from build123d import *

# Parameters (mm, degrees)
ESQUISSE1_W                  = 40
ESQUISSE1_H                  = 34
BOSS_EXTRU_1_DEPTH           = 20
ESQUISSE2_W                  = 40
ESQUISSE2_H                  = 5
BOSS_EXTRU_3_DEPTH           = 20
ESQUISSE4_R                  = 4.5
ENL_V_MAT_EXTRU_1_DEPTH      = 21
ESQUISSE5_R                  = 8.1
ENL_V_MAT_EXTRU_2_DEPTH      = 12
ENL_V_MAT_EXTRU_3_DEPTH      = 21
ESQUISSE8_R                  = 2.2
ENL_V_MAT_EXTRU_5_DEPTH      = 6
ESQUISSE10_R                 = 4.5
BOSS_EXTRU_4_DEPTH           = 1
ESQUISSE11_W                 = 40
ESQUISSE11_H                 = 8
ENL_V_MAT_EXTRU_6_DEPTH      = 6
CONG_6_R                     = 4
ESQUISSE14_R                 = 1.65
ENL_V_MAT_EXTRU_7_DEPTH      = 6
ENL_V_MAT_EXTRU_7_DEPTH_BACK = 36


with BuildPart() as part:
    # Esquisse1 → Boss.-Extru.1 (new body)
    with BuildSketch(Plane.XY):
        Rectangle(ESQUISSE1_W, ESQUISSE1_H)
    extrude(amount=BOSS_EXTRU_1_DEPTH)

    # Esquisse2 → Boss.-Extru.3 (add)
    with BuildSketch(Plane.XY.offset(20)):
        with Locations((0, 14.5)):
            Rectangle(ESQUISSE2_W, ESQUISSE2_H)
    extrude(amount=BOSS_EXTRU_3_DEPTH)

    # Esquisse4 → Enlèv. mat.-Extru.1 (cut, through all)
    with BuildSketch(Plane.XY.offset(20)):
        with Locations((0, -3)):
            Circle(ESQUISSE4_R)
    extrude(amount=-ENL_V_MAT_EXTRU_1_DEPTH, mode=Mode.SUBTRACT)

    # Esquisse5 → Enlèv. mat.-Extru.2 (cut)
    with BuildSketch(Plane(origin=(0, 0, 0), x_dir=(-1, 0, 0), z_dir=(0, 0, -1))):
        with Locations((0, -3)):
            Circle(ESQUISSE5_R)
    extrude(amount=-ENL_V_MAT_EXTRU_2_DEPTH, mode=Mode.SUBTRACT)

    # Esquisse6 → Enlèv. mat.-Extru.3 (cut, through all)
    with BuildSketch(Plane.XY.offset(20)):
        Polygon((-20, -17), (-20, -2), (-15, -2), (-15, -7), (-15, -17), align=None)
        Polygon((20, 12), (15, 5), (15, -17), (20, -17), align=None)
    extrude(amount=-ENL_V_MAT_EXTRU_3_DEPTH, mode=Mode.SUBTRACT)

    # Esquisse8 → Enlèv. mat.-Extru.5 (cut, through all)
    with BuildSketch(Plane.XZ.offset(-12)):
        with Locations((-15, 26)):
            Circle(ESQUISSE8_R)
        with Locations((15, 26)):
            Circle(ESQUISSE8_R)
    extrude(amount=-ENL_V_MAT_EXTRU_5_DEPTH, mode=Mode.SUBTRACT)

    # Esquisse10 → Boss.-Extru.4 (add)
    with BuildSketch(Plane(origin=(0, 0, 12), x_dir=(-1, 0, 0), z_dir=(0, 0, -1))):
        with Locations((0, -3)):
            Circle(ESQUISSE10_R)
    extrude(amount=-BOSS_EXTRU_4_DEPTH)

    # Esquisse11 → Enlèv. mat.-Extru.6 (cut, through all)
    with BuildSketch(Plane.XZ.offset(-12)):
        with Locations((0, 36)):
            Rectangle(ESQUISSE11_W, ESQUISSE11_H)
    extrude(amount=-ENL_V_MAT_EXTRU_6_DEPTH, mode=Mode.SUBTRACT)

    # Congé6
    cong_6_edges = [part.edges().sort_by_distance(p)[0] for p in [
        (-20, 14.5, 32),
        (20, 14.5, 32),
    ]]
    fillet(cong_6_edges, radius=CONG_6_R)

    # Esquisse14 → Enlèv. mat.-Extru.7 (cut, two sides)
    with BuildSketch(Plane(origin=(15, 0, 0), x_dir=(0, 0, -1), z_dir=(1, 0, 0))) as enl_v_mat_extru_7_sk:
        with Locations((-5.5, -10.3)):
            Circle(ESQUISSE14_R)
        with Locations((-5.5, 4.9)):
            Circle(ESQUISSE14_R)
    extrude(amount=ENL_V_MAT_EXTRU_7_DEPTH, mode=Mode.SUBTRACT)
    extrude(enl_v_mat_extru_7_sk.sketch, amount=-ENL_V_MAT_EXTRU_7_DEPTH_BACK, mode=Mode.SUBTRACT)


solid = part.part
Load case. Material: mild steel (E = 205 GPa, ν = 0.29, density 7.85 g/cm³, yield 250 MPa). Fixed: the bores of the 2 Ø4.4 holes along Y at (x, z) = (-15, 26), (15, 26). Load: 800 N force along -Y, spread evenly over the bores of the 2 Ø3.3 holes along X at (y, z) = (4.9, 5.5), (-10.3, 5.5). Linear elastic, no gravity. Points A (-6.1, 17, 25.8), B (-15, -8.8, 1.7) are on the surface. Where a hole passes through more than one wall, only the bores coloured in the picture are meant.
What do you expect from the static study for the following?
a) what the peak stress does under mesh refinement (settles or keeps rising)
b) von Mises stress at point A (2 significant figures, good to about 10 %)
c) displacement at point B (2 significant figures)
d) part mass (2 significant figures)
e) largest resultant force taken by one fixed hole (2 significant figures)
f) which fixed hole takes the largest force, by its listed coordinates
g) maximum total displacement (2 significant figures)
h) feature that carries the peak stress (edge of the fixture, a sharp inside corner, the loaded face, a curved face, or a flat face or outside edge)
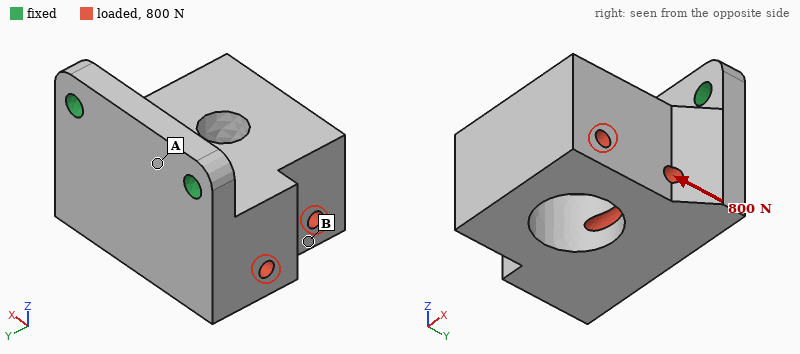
keeps rising
32 MPa
45 µm
170 g
440 N
(-15, 26)
56 µm
edge of the fixture
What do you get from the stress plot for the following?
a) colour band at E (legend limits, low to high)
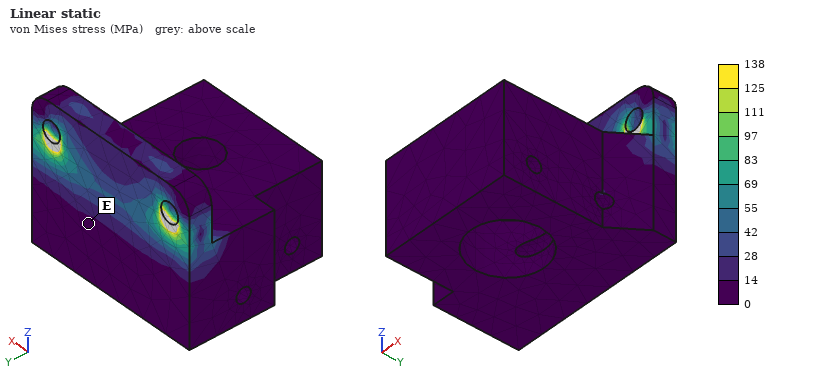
0 to 14 MPa
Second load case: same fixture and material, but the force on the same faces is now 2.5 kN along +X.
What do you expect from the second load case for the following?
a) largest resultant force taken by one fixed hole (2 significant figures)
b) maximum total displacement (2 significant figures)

2.4 kN
15 µm
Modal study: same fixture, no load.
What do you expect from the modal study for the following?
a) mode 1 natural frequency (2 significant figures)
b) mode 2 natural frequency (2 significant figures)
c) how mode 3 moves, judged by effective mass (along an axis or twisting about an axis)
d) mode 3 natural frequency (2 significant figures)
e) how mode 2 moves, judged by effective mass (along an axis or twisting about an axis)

1800 Hz
6600 Hz
along Y
11 kHz
along X
